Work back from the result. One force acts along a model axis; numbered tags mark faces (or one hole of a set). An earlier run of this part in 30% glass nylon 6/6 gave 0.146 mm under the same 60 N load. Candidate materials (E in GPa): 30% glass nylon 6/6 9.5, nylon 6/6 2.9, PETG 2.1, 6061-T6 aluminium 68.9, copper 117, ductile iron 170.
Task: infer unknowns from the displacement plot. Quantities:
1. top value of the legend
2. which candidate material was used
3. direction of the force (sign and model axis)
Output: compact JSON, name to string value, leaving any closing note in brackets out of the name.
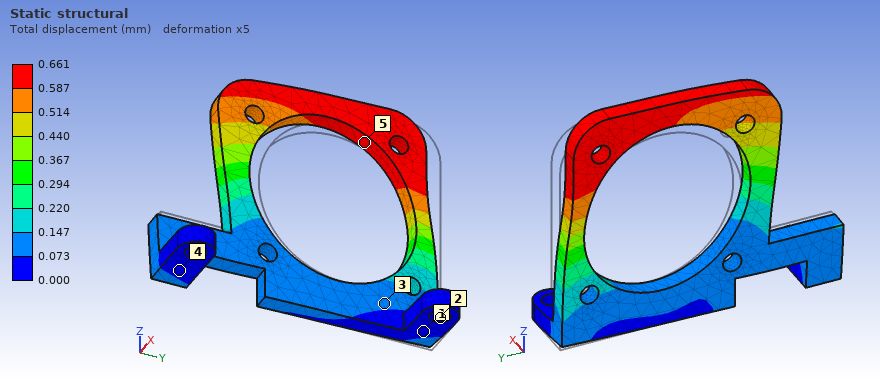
{"top value of the legend": "0.661 mm", "which candidate material was used": "PETG", "direction of the force": "-Y"}
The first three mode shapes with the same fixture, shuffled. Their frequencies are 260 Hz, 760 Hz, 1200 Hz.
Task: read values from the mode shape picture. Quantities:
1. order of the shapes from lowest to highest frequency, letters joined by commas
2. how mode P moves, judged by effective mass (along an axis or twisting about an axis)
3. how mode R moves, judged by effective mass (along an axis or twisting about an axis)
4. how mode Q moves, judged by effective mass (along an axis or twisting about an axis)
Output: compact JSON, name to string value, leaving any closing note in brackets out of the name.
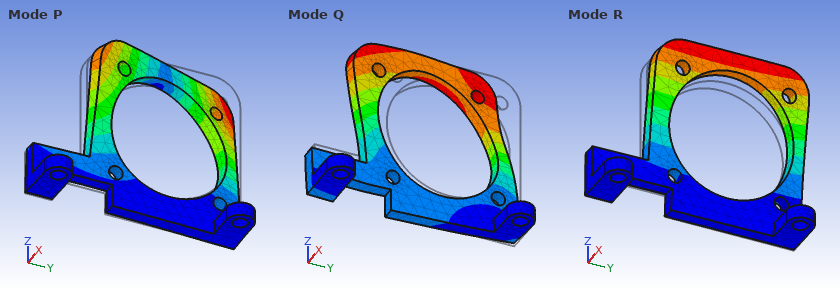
{"order of the shapes from lowest to highest frequency, letters joined by commas": "R, P, Q", "how mode P moves, judged by effective mass": "twisting about Z", "how mode R moves, judged by effective mass": "along X", "how mode Q moves, judged by effective mass": "along Y"}
